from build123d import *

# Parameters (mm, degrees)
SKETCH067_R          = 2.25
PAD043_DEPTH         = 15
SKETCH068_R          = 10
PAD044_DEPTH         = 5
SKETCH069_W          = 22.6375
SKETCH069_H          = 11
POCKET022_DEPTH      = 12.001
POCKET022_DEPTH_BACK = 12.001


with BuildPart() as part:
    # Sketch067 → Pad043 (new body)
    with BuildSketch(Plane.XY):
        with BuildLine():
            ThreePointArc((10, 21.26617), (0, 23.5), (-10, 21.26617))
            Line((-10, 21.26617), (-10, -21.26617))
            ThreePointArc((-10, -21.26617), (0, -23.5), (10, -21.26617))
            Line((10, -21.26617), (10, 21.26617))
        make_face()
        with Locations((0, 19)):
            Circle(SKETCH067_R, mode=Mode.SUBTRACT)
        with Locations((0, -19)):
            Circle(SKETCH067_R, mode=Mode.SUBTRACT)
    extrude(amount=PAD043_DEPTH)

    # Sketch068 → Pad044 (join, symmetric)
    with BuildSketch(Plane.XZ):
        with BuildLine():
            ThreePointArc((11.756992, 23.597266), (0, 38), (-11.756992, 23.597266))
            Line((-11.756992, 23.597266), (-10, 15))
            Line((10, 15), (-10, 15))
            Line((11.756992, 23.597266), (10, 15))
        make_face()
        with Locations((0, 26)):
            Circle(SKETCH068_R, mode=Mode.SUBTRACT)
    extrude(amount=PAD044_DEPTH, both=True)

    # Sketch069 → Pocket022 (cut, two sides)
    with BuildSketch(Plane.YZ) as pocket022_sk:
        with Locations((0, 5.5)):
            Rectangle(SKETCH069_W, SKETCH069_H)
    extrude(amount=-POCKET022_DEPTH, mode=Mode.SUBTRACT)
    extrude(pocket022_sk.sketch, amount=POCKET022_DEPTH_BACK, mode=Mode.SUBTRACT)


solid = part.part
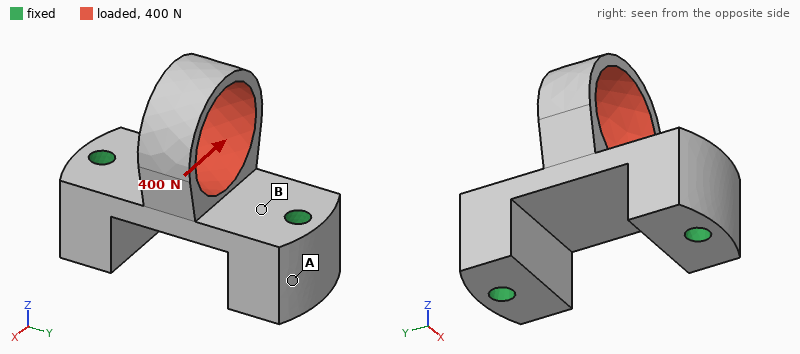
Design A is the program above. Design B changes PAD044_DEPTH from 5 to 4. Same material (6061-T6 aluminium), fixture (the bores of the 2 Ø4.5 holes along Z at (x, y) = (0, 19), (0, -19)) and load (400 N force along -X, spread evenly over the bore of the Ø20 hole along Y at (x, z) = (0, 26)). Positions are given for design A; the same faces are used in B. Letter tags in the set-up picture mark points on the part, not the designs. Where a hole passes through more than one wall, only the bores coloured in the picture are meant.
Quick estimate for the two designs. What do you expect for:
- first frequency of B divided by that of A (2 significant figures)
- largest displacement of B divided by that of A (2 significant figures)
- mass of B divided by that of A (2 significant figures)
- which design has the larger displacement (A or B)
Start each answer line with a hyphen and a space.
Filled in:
- 1.0
- 1.2
- 0.97
- B
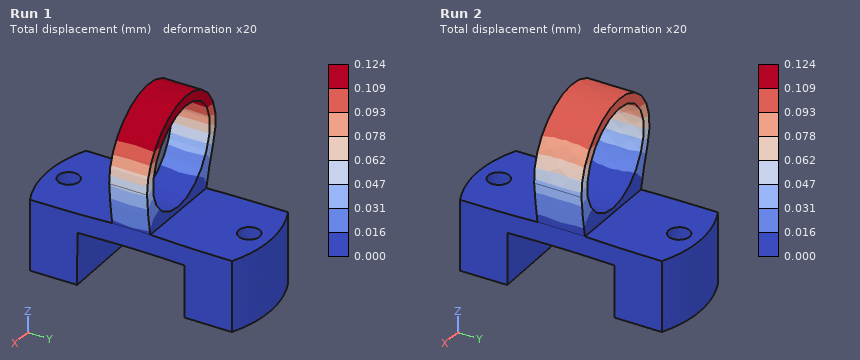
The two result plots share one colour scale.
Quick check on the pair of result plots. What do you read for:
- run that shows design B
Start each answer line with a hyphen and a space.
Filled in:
- Run 1
